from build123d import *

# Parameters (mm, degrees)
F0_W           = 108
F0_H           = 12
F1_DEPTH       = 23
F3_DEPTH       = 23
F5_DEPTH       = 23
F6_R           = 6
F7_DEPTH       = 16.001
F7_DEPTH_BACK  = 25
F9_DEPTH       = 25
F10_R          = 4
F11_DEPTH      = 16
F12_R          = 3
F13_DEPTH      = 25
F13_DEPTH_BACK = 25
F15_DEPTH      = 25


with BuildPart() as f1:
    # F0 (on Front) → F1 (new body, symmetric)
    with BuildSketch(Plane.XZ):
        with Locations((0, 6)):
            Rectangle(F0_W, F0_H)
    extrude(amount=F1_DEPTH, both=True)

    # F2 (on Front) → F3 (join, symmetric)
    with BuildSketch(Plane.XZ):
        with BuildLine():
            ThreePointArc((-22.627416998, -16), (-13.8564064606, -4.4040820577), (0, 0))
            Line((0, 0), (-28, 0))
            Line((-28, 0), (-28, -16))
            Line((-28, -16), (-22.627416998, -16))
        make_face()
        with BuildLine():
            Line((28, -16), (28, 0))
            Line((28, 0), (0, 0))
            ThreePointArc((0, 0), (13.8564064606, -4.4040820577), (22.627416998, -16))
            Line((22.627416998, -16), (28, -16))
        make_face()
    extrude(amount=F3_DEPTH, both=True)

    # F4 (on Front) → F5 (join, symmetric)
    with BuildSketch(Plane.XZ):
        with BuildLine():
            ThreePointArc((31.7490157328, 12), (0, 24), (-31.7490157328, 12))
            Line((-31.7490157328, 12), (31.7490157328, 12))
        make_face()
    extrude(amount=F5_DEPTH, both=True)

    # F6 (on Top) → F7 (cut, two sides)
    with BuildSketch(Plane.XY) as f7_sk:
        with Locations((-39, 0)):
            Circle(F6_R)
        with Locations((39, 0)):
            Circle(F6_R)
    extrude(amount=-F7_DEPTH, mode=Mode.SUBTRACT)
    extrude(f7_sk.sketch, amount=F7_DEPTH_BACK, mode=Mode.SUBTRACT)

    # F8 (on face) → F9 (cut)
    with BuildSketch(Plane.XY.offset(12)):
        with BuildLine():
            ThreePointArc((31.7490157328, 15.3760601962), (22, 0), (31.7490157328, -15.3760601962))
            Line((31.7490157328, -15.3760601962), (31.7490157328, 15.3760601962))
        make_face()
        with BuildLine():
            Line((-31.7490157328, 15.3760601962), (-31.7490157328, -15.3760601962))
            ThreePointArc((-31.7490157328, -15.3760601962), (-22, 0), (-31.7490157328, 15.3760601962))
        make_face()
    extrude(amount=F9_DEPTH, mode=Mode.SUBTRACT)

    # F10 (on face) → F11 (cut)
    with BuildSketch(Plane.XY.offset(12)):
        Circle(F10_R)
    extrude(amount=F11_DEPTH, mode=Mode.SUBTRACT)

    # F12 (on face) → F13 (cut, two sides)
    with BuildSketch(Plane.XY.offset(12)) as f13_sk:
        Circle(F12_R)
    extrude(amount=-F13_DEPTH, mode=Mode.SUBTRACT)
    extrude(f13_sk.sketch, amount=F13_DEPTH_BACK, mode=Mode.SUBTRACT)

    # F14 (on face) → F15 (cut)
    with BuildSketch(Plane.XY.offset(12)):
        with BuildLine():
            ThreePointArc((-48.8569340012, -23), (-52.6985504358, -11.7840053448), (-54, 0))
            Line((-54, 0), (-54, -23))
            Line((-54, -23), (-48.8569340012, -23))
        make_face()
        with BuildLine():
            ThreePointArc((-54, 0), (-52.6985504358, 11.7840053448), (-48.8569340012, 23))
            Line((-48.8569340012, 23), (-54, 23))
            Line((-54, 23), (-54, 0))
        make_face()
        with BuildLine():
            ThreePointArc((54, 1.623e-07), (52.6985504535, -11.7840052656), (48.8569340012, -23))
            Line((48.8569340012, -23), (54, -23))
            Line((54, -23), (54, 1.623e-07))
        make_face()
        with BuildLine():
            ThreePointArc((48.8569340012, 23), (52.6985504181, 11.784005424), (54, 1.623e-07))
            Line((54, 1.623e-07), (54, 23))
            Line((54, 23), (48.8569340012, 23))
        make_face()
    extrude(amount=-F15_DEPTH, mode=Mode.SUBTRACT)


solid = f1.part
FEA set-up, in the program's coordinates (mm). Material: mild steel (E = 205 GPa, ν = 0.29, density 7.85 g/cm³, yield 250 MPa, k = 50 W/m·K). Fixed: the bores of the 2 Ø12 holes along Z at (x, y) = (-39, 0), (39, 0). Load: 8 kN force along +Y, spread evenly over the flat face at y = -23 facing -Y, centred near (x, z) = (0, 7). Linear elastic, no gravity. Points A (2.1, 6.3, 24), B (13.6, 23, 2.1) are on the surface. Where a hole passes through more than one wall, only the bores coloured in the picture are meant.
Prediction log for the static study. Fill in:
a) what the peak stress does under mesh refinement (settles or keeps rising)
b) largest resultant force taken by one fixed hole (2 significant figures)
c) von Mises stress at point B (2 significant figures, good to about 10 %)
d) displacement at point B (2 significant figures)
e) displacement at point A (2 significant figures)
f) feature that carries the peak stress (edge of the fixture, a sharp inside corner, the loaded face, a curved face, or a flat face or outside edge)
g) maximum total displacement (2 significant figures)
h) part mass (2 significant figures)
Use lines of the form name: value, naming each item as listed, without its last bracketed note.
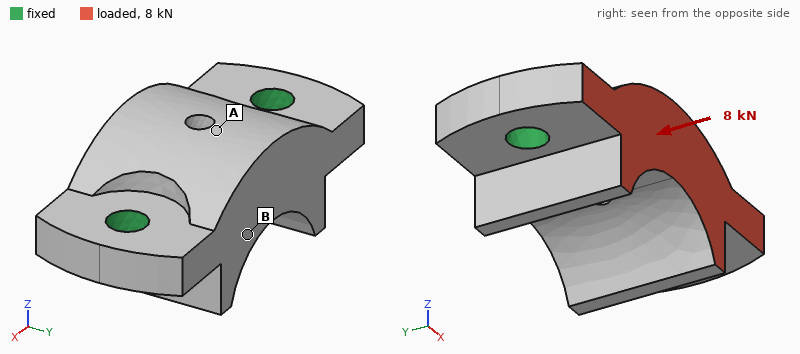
what the peak stress does under mesh refinement: keeps rising
largest resultant force taken by one fixed hole: 4.0 kN
von Mises stress at point B: 7.7 MPa
displacement at point B: 1.8 µm
displacement at point A: 2.8 µm
feature that carries the peak stress: edge of the fixture
maximum total displacement: 3.5 µm
part mass: 740 g
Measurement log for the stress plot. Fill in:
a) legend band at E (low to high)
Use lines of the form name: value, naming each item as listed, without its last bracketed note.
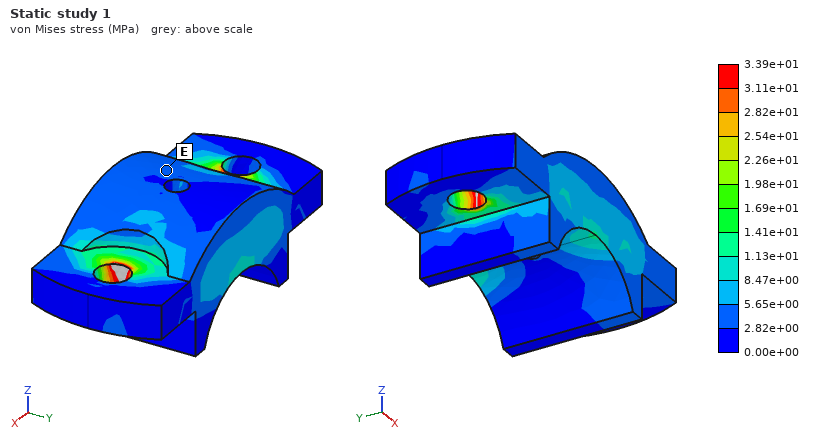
legend band at E: 2.82e+00 to 5.65e+00 MPa
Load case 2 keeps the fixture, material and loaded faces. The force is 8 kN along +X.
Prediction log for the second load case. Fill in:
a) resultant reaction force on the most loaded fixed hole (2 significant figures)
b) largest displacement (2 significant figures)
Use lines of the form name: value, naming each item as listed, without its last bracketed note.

resultant reaction force on the most loaded fixed hole: 4.5 kN
largest displacement: 3.5 µm
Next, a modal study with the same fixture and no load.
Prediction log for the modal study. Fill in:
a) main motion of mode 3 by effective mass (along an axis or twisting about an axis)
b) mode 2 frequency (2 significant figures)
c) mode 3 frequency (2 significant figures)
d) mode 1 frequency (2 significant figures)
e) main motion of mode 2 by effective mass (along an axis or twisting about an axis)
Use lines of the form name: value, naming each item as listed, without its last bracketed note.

main motion of mode 3 by effective mass: along Y
mode 2 frequency: 9200 Hz
mode 3 frequency: 12 kHz
mode 1 frequency: 7500 Hz
main motion of mode 2 by effective mass: along Z
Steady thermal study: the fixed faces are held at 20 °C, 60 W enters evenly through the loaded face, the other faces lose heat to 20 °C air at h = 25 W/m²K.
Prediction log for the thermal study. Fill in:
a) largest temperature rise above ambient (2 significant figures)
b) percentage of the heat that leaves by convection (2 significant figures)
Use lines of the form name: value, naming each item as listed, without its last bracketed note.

largest temperature rise above ambient: 26 K
percentage of the heat that leaves by convection: 7.3 %
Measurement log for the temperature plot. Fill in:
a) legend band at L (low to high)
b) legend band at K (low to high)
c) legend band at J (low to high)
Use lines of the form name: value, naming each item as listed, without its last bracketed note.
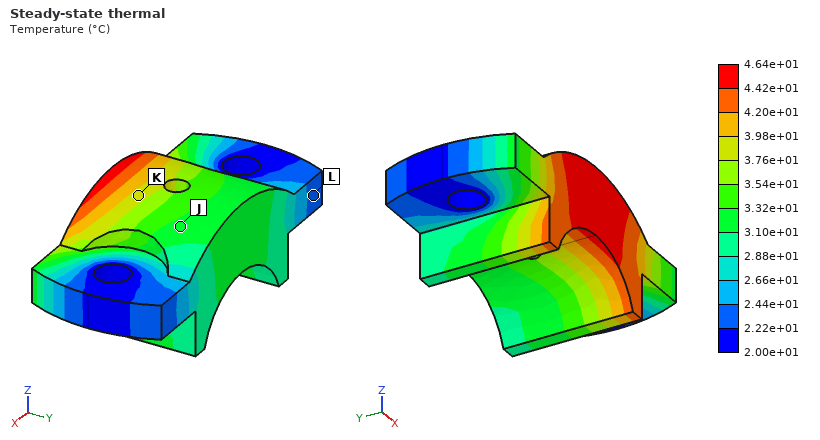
legend band at L: 2.22e+01 to 2.44e+01 °C
legend band at K: 3.76e+01 to 3.98e+01 °C
legend band at J: 3.10e+01 to 3.32e+01 °C
